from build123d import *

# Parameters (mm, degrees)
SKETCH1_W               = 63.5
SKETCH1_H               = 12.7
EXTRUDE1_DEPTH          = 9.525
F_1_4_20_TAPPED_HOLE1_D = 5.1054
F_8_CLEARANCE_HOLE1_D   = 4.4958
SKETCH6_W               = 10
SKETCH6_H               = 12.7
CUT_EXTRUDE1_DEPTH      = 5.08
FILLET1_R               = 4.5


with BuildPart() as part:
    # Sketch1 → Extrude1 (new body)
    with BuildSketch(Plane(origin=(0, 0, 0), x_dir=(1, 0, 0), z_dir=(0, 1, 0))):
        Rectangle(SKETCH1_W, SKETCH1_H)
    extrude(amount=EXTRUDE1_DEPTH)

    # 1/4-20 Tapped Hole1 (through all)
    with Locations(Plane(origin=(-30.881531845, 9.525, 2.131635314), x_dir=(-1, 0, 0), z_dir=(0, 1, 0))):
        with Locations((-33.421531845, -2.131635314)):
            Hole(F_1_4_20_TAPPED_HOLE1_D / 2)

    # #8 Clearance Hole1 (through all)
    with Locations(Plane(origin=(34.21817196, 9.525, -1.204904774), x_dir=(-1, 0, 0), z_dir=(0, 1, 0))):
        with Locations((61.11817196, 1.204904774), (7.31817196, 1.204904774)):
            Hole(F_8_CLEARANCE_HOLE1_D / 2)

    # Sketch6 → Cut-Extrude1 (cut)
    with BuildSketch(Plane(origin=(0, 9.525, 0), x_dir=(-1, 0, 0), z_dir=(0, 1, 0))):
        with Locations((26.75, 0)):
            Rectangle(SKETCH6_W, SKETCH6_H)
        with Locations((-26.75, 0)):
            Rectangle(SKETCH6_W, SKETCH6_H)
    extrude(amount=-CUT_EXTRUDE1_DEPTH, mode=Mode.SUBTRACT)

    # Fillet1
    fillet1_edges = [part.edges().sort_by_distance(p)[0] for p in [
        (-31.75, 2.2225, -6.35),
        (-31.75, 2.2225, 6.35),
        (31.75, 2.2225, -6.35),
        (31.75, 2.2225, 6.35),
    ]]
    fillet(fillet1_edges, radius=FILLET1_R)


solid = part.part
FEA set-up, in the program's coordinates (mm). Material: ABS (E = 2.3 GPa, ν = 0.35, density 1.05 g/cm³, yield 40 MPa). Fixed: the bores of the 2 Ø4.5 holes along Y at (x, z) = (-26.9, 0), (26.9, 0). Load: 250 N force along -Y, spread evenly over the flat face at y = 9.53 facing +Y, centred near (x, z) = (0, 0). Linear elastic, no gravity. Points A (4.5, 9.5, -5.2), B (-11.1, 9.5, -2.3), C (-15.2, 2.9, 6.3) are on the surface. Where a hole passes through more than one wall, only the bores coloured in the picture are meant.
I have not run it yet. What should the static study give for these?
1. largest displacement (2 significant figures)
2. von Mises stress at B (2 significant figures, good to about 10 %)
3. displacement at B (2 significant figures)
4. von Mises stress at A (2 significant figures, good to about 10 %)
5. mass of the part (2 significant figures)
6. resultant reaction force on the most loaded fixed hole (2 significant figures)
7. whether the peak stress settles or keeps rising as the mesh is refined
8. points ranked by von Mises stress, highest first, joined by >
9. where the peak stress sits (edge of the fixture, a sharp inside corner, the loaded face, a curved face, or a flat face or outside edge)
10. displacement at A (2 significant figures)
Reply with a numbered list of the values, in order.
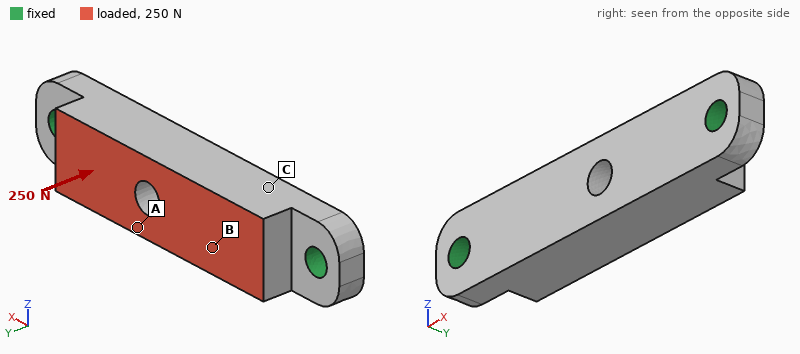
1. 0.15 mm
2. 4.0 MPa
3. 0.11 mm
4. 7.8 MPa
5. 6.3 g
6. 180 N
7. keeps rising
8. A > B > C
9. edge of the fixture
10. 0.14 mm
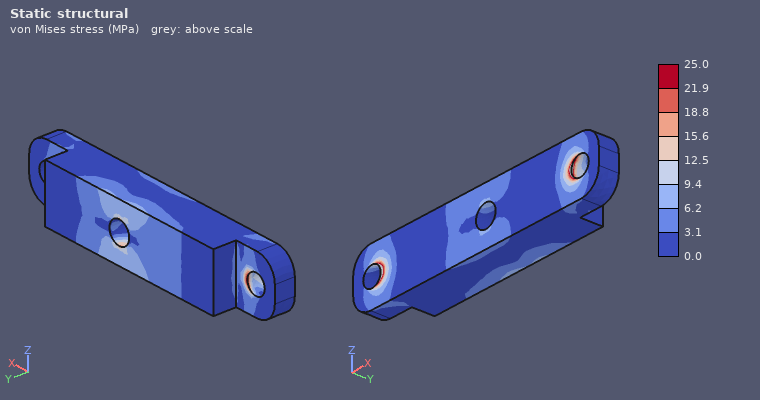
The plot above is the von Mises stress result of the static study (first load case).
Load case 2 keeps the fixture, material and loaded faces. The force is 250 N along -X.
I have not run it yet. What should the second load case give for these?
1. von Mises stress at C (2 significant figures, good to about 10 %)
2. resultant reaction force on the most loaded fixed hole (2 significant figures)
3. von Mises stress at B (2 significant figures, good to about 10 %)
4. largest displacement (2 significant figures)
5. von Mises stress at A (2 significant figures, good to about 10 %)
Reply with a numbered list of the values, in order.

1. 1.2 MPa
2. 130 N
3. 0.83 MPa
4. 19 µm
5. 0.86 MPa
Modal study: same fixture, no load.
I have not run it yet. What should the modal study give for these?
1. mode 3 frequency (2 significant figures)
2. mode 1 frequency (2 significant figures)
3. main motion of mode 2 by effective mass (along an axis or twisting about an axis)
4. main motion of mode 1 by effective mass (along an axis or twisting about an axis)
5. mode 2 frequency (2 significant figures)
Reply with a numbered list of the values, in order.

1. 5100 Hz
2. 3200 Hz
3. along Z
4. along Y
5. 3400 Hz
